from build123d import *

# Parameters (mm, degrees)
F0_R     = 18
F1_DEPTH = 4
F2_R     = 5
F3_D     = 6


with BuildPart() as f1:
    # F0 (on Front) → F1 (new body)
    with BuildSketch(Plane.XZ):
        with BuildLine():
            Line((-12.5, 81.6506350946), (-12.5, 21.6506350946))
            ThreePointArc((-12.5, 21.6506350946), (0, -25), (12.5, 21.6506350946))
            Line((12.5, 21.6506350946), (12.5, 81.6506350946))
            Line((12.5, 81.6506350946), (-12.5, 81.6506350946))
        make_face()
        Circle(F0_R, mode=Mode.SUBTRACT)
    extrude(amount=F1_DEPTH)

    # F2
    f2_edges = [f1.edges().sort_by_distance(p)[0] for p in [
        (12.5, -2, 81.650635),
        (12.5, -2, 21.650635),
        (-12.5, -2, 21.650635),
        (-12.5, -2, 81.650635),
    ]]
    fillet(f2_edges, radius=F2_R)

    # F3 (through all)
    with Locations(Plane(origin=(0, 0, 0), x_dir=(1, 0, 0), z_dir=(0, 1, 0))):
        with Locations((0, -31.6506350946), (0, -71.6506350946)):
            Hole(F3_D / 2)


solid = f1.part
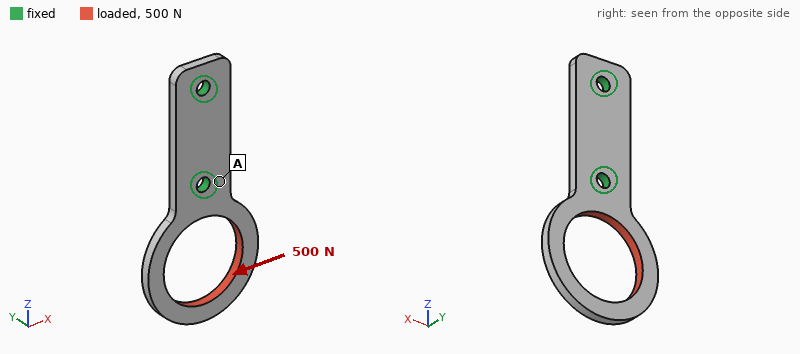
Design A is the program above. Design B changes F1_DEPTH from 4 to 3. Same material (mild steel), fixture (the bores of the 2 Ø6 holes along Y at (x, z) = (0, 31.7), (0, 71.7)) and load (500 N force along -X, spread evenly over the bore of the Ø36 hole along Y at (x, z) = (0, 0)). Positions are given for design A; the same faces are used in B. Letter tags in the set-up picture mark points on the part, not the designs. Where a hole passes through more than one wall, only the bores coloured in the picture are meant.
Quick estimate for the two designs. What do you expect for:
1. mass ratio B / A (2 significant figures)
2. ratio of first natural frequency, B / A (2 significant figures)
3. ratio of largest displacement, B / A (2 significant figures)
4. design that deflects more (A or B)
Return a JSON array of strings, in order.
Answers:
["0.75", "0.77", "1.3", "B"]
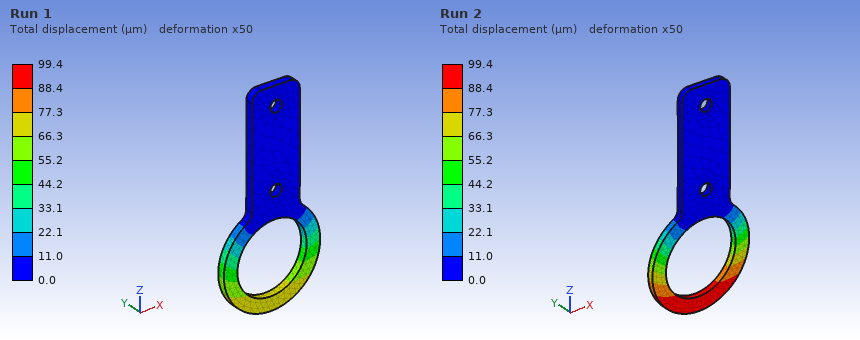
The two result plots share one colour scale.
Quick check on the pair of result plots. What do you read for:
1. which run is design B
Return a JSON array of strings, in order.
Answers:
["Run 2"]
